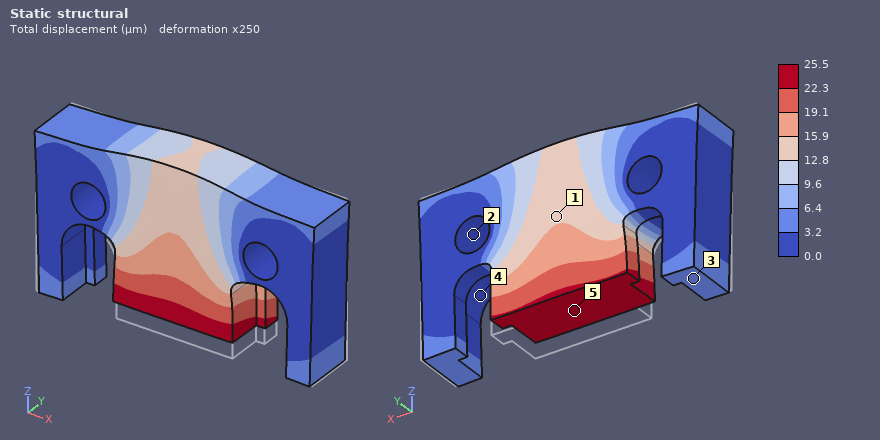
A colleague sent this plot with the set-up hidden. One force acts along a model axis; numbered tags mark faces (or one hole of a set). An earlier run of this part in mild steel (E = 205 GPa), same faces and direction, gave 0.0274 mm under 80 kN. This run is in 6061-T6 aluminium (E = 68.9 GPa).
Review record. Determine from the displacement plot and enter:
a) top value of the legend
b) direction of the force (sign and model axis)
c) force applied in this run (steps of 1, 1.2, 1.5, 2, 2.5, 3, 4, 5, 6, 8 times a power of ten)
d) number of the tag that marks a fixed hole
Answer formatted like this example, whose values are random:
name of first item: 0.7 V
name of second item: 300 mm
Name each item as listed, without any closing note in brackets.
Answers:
top value of the legend: 25.5 µm
direction of the force: +Z
force applied in this run: 25 kN
number of the tag that marks a fixed hole: 2
